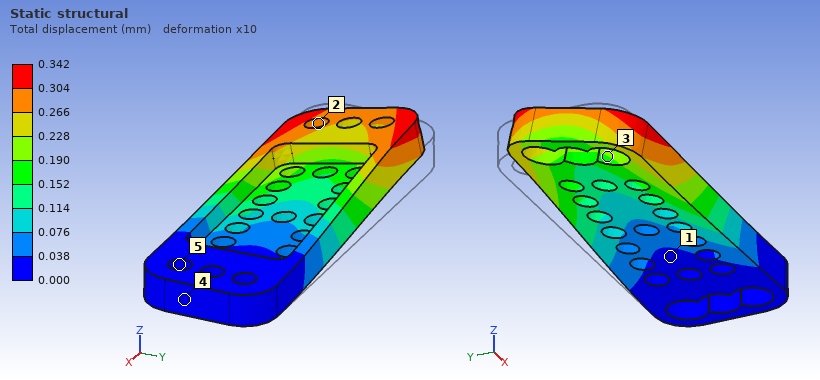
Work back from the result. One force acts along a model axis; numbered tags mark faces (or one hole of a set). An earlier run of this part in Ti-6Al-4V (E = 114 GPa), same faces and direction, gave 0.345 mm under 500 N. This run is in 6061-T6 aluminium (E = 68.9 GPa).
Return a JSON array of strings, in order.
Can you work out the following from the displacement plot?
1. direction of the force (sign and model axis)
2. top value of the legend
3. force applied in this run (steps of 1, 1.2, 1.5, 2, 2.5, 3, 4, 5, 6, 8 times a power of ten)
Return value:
["-Y", "0.342 mm", "300 N"]
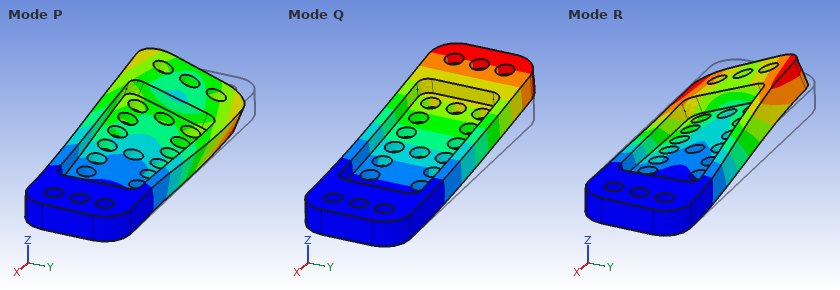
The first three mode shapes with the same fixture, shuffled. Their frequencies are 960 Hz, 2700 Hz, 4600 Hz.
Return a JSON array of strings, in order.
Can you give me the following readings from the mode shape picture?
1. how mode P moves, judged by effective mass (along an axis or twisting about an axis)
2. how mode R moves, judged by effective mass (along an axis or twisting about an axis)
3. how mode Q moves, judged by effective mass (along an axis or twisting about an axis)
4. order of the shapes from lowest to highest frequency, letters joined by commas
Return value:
["along Y", "along Y", "along Z", "Q, R, P"]
